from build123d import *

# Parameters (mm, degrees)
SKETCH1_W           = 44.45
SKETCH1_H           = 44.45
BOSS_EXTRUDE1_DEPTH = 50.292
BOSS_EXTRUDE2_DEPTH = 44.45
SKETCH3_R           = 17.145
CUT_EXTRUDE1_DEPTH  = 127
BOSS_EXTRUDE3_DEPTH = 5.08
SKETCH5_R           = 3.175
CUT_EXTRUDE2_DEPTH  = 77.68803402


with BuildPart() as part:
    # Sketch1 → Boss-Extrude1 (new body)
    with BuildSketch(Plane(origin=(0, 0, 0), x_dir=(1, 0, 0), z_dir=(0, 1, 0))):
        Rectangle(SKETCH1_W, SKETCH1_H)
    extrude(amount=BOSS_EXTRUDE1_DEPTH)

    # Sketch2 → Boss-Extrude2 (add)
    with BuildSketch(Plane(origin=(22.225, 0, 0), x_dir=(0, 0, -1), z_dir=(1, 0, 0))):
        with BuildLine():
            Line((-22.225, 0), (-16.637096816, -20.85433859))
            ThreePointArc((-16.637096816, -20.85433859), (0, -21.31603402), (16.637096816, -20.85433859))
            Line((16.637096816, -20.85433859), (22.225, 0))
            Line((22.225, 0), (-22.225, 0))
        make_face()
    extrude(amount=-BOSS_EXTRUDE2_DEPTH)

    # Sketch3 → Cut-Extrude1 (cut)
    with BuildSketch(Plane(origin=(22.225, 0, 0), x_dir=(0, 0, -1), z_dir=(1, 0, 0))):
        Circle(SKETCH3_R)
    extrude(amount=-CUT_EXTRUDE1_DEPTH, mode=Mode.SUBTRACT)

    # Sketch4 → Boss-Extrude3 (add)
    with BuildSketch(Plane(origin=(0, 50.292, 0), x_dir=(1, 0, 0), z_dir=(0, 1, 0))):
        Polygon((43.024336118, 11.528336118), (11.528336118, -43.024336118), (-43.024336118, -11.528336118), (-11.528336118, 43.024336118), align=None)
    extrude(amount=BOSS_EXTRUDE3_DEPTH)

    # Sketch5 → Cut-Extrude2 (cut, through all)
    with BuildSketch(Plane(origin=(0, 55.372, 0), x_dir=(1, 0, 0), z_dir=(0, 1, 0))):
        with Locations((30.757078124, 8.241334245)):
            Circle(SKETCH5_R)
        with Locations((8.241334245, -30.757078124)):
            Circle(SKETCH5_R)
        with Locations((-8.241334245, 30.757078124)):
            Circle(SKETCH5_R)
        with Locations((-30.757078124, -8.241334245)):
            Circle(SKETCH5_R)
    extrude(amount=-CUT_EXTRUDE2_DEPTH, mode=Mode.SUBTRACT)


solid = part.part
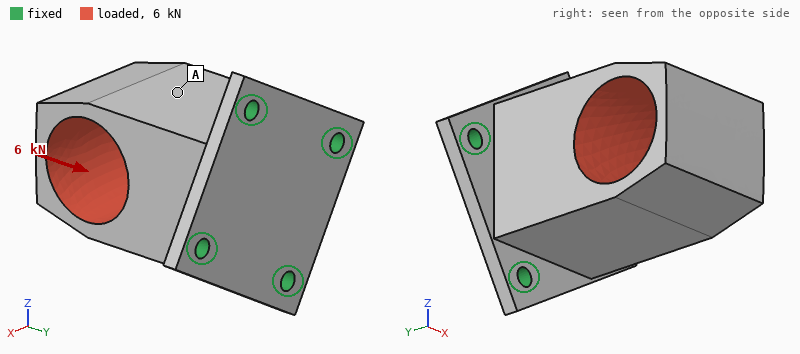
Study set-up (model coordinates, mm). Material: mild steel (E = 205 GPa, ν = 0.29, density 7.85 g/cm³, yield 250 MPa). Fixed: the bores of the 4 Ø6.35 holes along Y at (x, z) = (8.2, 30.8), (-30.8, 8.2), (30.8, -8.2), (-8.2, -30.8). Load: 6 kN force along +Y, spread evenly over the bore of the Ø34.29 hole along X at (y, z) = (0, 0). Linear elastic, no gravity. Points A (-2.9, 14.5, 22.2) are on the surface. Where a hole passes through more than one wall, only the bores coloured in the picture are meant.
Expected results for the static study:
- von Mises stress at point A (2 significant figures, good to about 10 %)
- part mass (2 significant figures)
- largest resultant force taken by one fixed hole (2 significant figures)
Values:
12 MPa
900 g
1.6 kN
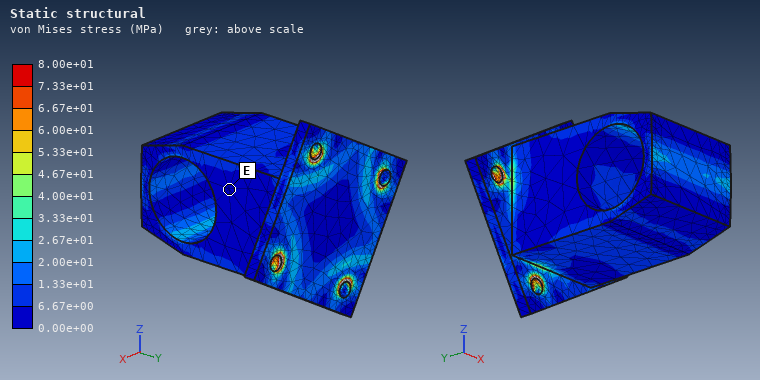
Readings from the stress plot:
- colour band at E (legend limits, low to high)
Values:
0.00e+00 to 6.67e+00 MPa
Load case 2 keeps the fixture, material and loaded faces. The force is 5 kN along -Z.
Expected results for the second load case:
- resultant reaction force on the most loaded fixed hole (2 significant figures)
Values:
4.9 kN
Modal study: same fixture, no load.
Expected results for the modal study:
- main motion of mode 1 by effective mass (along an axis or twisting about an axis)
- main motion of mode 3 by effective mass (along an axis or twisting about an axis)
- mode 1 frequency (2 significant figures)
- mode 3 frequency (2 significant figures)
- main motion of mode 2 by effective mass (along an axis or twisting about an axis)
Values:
along Z
along Y
2900 Hz
6000 Hz
along X
